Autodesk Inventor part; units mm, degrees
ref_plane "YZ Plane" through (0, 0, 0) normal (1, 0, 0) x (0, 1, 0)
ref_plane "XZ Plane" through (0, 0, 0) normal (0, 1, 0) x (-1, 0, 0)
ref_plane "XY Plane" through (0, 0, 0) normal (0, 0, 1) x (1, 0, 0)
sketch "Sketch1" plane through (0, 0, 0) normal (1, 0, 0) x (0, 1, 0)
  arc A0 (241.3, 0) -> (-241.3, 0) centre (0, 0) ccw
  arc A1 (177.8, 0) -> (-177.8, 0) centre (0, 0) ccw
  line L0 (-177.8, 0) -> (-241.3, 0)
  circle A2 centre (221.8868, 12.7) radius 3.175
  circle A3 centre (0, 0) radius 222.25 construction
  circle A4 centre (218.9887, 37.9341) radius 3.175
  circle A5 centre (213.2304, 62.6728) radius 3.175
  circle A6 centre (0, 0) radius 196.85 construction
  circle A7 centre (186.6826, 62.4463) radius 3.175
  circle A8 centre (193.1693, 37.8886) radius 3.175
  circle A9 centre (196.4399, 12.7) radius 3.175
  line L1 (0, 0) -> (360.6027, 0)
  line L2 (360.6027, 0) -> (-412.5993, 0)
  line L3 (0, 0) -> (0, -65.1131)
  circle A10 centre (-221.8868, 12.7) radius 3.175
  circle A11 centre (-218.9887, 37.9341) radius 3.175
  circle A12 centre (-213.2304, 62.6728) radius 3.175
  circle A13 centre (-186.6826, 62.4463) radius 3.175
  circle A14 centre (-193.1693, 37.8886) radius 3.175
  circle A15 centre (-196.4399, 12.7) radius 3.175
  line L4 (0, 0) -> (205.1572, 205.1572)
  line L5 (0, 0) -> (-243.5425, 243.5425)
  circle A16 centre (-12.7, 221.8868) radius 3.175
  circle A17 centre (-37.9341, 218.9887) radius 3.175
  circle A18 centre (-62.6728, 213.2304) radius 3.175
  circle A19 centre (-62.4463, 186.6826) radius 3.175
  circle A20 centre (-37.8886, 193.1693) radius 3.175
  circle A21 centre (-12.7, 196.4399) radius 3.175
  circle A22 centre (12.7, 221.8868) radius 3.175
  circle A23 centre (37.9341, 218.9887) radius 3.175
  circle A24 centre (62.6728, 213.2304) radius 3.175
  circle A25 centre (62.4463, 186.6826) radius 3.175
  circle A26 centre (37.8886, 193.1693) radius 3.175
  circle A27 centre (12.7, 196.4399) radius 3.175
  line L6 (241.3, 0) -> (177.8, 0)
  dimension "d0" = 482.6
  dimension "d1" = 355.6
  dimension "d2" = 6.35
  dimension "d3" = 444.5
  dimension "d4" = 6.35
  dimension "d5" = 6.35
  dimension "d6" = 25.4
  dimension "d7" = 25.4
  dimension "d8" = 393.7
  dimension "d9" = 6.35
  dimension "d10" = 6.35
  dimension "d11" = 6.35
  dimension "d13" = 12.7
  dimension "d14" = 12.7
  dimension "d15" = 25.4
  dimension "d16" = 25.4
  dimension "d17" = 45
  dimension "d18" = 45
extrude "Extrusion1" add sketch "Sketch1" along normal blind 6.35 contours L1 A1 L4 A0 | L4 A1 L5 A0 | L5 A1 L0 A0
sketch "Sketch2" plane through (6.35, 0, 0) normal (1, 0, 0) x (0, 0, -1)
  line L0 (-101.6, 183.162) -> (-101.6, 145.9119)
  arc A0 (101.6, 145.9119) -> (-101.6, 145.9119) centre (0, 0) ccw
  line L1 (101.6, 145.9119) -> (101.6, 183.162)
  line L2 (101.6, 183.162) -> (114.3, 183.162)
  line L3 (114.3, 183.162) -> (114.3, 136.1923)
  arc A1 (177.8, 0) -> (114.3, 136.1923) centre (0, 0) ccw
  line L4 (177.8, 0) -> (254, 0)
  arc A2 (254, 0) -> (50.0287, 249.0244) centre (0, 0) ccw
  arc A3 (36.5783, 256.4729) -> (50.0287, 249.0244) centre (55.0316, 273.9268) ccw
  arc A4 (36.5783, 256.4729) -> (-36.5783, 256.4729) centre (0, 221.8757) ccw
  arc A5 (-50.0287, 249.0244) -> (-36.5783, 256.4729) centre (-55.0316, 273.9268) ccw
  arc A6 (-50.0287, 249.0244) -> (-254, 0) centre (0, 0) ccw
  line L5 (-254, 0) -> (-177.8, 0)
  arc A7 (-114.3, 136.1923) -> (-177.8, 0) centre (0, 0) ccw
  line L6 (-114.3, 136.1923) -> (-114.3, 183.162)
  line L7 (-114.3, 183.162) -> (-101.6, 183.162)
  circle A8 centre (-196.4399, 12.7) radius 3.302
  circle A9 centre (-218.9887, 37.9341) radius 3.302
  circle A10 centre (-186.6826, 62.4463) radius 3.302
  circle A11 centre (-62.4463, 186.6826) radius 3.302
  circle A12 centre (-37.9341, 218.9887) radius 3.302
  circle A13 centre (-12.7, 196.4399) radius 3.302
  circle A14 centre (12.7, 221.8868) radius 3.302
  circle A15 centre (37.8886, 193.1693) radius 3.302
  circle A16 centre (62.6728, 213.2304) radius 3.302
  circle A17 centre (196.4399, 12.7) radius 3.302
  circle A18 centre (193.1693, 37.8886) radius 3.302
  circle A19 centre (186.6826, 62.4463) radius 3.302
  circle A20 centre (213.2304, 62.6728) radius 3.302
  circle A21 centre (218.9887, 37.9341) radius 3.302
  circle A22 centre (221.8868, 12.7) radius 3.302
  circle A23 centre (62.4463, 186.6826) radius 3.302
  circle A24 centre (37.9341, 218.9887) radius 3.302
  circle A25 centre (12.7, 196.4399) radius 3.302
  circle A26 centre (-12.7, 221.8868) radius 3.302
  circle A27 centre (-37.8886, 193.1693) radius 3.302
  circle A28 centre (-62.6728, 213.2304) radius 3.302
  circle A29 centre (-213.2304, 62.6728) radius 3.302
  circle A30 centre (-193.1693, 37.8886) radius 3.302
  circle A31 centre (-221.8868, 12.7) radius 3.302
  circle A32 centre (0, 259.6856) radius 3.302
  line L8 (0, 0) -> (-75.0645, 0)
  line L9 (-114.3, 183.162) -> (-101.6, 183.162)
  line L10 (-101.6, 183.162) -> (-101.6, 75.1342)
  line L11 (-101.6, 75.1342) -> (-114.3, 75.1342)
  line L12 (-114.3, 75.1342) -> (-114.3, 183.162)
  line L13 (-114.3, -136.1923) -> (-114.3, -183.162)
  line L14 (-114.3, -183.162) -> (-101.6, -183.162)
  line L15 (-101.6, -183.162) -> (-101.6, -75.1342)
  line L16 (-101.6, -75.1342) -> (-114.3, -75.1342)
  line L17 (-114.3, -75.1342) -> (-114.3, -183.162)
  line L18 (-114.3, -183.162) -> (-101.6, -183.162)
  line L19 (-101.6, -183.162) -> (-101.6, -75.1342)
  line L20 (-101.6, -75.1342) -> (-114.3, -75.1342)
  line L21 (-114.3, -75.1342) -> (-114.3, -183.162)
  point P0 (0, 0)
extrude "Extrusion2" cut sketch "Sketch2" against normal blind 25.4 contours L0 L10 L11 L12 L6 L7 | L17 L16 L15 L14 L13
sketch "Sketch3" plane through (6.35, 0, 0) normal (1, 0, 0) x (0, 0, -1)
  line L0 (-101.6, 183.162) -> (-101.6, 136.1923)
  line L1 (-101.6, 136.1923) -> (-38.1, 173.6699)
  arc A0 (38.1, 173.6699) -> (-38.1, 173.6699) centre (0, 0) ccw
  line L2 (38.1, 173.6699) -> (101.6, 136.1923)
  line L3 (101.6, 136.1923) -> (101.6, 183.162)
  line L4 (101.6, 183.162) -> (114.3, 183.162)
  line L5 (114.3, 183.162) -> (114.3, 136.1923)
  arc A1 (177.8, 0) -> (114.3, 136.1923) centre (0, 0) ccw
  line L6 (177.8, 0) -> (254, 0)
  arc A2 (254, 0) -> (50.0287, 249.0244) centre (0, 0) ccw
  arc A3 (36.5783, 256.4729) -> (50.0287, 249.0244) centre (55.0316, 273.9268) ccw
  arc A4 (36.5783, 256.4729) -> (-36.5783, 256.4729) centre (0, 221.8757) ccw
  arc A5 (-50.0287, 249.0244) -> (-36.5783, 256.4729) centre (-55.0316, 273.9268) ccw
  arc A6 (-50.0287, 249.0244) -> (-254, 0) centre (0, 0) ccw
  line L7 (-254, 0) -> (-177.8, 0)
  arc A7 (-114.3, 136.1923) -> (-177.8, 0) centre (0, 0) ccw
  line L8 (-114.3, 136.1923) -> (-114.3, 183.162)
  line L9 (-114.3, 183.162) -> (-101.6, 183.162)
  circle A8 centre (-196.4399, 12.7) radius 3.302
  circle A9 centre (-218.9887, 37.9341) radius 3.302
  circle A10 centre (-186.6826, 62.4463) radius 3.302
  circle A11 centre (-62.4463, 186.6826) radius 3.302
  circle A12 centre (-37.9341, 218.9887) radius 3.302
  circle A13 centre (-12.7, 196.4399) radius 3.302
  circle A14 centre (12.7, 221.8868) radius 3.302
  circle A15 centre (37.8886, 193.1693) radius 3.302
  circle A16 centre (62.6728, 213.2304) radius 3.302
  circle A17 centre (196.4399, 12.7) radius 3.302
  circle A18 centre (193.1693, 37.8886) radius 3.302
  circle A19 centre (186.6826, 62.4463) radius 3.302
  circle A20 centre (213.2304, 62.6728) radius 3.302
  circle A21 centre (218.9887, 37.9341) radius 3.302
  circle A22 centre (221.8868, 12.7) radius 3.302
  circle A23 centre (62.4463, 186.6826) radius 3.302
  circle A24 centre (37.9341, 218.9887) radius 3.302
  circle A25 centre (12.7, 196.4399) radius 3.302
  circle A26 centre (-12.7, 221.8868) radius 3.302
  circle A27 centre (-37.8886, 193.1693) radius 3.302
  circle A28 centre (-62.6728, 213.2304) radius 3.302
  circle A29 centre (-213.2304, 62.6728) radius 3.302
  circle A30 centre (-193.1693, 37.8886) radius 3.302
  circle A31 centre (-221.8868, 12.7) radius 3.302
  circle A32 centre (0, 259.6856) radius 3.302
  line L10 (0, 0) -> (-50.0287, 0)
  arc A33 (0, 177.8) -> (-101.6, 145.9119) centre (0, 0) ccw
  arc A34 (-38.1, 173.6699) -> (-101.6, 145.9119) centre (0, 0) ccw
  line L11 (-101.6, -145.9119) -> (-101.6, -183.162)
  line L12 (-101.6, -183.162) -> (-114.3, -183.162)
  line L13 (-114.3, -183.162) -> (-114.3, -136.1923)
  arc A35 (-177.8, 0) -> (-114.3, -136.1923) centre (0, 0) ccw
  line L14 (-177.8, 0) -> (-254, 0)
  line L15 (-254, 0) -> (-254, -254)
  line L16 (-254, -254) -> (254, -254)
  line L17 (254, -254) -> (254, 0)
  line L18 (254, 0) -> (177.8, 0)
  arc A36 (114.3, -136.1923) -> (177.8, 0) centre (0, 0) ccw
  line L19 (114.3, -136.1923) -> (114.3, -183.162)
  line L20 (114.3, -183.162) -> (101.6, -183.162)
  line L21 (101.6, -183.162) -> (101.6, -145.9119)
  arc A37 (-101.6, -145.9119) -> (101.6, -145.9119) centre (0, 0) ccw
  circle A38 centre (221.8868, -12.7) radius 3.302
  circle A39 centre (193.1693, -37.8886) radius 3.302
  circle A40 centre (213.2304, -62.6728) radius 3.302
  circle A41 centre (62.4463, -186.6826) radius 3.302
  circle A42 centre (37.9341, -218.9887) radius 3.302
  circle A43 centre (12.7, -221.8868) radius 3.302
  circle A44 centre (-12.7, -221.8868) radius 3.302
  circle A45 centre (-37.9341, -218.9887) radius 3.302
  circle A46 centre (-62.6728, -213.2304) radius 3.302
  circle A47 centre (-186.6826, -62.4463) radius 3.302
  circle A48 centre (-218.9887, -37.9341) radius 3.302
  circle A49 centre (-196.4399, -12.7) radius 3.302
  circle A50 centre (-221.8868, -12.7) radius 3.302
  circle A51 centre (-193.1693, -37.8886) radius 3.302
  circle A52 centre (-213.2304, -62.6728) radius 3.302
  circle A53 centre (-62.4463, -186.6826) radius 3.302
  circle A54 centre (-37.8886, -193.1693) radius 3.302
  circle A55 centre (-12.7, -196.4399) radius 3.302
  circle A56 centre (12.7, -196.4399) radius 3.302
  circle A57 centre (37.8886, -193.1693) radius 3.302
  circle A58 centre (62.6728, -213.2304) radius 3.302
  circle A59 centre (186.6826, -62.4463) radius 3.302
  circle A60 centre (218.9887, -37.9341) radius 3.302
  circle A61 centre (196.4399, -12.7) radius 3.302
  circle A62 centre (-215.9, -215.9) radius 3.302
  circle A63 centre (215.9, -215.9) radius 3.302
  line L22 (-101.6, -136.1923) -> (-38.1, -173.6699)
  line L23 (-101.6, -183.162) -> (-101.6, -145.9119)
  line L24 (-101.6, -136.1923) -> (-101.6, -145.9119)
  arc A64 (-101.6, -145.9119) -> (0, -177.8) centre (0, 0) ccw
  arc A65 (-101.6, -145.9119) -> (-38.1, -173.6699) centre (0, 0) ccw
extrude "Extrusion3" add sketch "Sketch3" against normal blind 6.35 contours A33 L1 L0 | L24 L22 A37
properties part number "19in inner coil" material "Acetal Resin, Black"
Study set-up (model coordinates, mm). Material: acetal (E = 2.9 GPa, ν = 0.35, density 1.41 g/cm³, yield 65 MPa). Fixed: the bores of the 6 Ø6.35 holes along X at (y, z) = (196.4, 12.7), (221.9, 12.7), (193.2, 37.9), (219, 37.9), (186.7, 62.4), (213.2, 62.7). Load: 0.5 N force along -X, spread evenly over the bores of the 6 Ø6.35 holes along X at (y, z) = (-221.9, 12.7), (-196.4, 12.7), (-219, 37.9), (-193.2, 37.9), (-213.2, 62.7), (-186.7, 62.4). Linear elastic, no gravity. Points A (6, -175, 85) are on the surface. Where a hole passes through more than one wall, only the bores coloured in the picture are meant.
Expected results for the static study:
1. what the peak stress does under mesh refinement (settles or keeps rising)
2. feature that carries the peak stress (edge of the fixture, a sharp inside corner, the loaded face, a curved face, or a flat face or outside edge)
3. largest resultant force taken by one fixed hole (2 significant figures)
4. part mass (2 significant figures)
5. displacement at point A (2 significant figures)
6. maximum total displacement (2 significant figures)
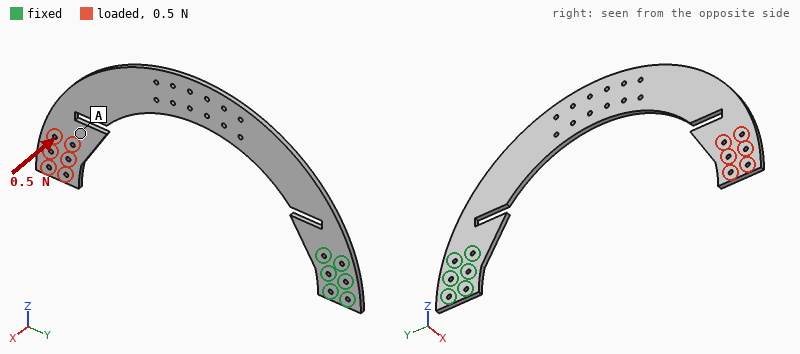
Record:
keeps rising
a sharp inside corner
6.8 N
370 g
4.5 mm
6.0 mm
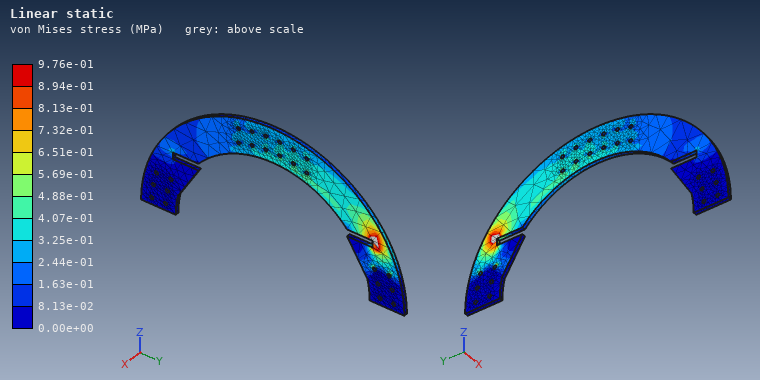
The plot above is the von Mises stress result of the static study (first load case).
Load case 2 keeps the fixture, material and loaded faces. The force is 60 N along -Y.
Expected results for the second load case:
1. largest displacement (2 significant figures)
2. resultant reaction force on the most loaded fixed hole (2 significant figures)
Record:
6.1 mm
44 N
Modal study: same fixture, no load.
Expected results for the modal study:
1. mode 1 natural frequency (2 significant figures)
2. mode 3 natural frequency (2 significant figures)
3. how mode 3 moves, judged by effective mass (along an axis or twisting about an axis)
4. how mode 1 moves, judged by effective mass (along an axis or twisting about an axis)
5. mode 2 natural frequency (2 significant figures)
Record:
4.7 Hz
26 Hz
along Z
along X
15 Hz
